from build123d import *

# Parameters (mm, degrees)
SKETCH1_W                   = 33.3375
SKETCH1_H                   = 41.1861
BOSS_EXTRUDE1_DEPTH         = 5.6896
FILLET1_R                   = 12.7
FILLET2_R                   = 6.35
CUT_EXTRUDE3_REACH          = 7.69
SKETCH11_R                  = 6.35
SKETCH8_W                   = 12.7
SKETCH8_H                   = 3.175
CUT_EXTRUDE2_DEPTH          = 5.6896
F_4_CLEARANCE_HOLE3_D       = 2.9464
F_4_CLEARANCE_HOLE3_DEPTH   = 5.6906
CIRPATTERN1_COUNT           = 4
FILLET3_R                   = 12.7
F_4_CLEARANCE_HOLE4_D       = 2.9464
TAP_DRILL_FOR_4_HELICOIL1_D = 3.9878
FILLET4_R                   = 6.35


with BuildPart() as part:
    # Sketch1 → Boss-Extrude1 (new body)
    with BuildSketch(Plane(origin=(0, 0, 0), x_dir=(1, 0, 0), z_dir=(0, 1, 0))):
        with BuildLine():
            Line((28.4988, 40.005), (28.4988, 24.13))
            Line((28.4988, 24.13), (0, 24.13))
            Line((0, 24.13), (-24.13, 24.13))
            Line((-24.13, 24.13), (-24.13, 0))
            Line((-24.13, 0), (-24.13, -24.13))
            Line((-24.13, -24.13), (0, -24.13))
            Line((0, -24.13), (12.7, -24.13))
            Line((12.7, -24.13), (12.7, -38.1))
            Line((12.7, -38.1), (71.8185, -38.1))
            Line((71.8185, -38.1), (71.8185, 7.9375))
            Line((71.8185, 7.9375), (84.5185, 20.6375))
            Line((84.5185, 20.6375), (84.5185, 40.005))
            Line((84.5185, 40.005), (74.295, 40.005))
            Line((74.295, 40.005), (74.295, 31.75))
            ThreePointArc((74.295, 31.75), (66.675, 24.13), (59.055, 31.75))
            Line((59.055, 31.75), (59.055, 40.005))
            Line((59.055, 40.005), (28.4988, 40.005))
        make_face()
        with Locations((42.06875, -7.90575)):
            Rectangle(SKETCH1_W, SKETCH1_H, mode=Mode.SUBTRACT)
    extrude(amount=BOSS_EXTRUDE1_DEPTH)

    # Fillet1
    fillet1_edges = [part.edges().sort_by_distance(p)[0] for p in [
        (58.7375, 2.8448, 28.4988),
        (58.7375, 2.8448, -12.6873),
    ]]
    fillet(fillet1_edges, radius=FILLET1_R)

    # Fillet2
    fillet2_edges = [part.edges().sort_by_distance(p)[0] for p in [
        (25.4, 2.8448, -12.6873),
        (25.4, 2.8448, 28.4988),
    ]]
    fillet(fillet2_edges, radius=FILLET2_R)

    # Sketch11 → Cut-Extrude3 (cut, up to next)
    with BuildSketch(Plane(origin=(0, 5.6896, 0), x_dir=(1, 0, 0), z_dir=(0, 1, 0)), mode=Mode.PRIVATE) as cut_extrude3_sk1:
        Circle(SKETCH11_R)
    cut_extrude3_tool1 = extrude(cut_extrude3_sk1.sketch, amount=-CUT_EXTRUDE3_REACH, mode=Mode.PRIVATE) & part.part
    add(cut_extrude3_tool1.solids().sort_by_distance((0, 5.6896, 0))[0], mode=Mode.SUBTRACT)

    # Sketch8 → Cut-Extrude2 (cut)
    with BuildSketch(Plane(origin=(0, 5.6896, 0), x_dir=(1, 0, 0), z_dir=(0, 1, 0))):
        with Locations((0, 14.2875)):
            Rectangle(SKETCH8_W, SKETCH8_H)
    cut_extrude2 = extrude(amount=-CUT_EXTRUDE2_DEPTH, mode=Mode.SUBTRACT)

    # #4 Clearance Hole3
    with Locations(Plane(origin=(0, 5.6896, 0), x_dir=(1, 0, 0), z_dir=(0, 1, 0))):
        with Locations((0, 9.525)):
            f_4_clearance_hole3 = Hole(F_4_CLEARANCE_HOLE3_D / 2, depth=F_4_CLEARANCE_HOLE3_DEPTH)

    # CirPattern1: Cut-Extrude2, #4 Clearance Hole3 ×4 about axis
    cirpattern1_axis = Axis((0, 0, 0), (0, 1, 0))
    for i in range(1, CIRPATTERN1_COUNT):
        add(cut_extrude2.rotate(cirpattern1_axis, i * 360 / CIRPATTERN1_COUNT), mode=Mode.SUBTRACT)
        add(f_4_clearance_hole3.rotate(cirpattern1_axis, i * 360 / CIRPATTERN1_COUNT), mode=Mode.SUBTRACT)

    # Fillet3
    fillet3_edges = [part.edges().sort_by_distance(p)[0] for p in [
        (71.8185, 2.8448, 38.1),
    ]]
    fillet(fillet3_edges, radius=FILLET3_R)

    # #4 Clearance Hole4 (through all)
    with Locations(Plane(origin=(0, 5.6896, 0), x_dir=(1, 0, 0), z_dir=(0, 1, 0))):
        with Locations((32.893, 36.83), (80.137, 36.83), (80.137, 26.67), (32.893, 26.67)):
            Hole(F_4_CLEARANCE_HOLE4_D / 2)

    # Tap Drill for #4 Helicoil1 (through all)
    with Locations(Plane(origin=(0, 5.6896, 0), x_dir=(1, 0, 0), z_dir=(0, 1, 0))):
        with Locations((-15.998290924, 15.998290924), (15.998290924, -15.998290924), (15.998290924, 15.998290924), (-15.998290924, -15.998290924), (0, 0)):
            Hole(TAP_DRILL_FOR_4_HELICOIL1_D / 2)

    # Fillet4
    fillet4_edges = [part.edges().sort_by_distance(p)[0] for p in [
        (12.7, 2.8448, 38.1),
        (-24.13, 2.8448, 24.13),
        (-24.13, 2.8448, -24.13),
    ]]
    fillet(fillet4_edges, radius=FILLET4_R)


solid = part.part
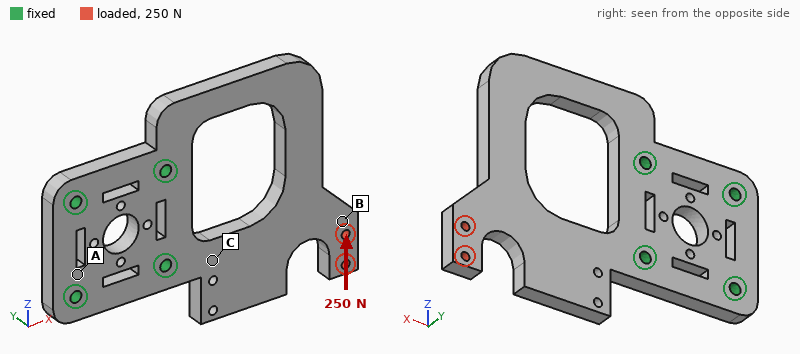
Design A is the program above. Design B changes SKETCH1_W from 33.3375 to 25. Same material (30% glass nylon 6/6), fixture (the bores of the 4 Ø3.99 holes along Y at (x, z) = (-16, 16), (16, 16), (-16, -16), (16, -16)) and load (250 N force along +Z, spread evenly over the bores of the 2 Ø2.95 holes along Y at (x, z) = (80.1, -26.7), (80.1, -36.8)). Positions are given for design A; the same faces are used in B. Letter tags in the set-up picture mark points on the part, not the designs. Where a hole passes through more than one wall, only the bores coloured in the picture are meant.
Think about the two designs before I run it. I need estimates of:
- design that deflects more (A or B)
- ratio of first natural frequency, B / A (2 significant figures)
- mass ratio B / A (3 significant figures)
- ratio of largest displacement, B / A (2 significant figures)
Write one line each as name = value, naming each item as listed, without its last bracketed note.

design that deflects more = A
ratio of first natural frequency, B / A = 1.1
mass ratio B / A = 1.08
ratio of largest displacement, B / A = 0.67
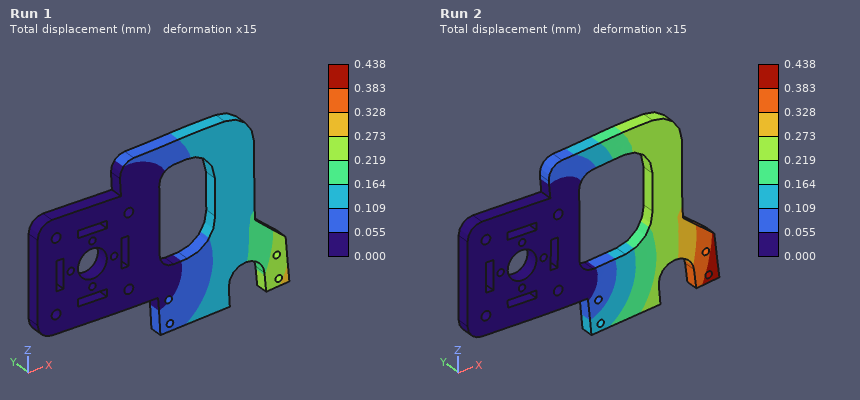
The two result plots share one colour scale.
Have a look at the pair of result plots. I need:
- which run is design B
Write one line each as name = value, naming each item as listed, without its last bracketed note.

which run is design B = Run 1
